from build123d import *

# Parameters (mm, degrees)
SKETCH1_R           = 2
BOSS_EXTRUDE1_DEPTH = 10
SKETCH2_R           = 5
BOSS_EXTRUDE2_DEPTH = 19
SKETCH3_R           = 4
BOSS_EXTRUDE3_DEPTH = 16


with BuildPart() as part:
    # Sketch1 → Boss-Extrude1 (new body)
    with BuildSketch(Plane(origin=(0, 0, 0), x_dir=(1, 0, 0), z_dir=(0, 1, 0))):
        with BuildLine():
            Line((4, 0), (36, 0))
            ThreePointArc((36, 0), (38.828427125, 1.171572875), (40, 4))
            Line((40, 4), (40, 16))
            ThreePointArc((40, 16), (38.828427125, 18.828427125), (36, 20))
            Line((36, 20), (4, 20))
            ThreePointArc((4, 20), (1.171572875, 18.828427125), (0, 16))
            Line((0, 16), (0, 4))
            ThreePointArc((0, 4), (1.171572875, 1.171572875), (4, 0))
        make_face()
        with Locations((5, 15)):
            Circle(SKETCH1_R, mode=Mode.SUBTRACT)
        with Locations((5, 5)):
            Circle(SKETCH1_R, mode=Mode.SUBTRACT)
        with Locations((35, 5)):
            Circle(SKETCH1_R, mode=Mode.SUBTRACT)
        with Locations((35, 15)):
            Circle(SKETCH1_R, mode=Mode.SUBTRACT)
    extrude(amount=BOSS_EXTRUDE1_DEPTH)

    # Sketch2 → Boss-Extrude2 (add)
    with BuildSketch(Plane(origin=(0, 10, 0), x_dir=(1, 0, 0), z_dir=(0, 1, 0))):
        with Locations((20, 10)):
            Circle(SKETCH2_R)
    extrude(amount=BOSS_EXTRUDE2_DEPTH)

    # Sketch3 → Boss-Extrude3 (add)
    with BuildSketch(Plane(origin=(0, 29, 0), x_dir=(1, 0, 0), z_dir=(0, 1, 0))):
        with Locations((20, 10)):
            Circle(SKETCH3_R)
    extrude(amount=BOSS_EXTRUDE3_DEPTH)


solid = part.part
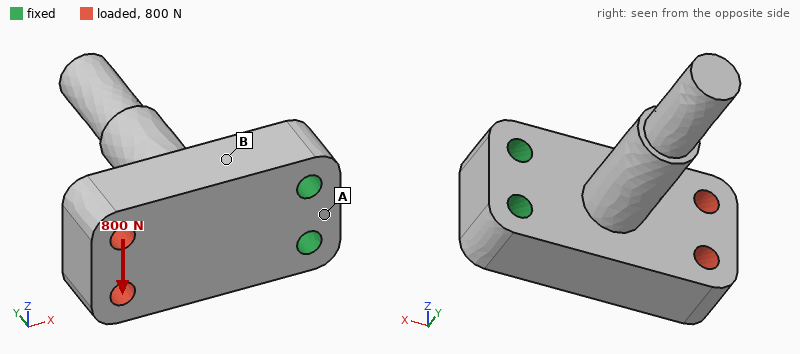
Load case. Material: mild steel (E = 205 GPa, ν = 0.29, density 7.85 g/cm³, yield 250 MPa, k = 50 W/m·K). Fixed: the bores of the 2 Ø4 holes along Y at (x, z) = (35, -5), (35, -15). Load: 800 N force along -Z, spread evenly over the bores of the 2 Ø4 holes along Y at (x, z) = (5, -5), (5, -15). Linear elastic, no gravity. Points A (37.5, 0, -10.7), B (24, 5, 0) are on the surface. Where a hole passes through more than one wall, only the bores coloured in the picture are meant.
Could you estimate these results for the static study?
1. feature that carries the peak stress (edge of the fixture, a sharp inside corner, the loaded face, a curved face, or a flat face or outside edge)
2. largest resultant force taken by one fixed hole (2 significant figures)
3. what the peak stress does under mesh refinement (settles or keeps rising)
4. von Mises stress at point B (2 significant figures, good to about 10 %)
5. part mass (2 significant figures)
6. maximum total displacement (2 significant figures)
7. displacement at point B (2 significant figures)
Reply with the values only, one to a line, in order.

edge of the fixture
1.9 kN
keeps rising
22 MPa
76 g
9.0 µm
2.5 µm
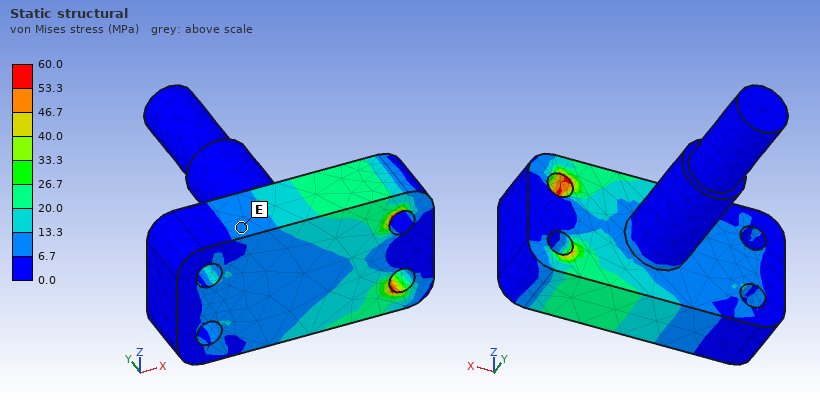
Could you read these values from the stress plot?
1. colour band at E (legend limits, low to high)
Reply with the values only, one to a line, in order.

6.7 to 13.3 MPa
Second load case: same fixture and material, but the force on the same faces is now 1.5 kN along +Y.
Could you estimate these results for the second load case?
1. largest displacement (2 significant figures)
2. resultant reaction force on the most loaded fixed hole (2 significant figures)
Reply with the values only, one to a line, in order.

59 µm
750 N
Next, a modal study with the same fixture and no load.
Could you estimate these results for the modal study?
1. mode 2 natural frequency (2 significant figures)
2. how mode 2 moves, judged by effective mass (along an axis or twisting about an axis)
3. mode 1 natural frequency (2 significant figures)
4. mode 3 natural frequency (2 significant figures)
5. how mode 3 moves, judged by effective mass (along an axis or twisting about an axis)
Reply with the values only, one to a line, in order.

5100 Hz
along Z
4400 Hz
8800 Hz
along Y
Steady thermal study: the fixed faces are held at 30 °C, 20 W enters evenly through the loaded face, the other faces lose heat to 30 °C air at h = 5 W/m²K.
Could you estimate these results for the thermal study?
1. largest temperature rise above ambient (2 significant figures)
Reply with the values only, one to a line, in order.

61 K
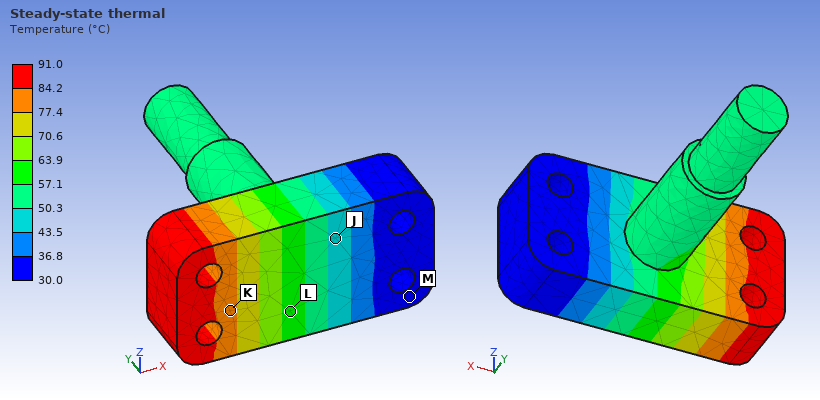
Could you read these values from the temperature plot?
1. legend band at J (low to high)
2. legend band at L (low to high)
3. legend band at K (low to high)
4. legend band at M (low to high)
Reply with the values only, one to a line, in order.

43.5 to 50.3 °C
57.1 to 63.9 °C
77.4 to 84.2 °C
30.0 to 36.8 °C
